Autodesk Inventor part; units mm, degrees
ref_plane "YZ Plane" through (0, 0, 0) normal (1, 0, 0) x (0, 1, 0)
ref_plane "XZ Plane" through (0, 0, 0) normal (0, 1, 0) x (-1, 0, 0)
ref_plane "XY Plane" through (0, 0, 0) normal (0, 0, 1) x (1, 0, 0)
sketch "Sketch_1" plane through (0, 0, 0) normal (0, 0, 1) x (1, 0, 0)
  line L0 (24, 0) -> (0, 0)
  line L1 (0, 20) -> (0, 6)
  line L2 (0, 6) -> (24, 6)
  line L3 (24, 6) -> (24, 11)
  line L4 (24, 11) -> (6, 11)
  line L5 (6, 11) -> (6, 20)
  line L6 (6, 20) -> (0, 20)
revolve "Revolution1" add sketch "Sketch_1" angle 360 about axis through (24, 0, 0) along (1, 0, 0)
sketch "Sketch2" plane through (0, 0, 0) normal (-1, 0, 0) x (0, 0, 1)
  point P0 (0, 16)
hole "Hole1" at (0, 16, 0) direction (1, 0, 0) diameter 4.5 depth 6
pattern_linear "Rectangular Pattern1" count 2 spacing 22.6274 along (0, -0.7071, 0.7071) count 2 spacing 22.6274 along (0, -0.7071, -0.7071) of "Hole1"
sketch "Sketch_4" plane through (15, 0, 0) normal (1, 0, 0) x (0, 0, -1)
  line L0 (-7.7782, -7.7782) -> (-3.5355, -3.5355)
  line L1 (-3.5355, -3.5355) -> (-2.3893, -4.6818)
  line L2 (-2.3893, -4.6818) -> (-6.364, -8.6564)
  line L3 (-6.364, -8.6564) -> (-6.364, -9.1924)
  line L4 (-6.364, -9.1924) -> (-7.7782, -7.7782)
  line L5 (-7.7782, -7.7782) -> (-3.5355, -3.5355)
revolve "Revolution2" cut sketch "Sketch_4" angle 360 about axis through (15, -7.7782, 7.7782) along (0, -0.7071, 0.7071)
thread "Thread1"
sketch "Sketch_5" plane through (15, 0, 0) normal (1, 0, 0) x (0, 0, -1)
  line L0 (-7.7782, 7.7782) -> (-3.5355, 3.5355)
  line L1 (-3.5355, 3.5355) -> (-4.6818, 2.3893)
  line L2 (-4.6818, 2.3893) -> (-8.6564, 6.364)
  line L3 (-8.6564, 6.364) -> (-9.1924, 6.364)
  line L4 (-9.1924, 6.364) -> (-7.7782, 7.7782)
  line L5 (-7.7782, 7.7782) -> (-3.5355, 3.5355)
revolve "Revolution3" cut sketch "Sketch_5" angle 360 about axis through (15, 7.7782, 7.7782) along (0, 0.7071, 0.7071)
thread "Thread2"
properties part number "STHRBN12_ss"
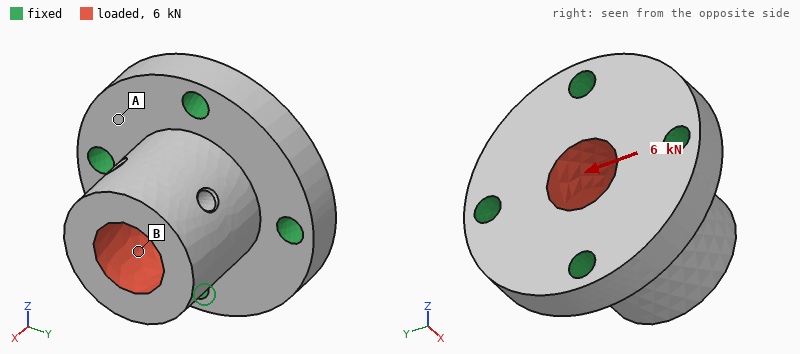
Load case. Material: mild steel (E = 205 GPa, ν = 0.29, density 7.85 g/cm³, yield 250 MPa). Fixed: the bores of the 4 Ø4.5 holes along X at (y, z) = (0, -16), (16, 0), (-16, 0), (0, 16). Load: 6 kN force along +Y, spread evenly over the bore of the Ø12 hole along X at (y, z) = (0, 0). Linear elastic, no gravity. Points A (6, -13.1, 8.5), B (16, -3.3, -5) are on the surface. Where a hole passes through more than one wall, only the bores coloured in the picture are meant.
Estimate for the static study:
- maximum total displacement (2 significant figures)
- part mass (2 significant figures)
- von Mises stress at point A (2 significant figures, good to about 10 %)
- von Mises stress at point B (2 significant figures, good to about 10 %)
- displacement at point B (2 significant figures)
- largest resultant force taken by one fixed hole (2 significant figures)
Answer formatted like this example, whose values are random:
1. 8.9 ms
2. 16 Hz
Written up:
1. 11 µm
2. 88 g
3. 13 MPa
4. 33 MPa
5. 6.7 µm
6. 2.6 kN
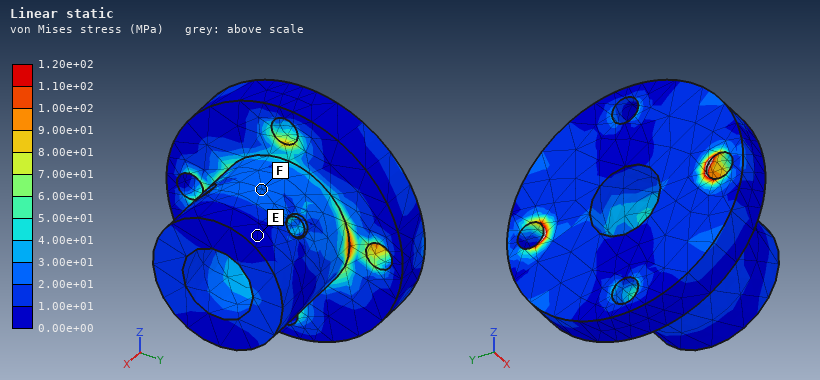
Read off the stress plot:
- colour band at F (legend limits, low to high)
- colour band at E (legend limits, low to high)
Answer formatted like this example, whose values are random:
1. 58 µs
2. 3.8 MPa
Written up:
1. 2.00e+01 to 3.00e+01 MPa
2. 0.00e+00 to 1.00e+01 MPa
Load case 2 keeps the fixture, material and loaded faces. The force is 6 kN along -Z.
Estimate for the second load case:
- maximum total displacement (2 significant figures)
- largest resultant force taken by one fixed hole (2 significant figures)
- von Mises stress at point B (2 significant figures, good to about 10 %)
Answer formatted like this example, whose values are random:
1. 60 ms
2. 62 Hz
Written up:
1. 11 µm
2. 2.6 kN
3. 25 MPa
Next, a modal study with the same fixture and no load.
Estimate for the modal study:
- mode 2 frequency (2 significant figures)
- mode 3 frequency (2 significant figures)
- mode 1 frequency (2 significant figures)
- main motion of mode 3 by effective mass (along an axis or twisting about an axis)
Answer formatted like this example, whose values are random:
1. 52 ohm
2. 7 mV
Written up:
1. 19 kHz
2. 31 kHz
3. 19 kHz
4. along X
